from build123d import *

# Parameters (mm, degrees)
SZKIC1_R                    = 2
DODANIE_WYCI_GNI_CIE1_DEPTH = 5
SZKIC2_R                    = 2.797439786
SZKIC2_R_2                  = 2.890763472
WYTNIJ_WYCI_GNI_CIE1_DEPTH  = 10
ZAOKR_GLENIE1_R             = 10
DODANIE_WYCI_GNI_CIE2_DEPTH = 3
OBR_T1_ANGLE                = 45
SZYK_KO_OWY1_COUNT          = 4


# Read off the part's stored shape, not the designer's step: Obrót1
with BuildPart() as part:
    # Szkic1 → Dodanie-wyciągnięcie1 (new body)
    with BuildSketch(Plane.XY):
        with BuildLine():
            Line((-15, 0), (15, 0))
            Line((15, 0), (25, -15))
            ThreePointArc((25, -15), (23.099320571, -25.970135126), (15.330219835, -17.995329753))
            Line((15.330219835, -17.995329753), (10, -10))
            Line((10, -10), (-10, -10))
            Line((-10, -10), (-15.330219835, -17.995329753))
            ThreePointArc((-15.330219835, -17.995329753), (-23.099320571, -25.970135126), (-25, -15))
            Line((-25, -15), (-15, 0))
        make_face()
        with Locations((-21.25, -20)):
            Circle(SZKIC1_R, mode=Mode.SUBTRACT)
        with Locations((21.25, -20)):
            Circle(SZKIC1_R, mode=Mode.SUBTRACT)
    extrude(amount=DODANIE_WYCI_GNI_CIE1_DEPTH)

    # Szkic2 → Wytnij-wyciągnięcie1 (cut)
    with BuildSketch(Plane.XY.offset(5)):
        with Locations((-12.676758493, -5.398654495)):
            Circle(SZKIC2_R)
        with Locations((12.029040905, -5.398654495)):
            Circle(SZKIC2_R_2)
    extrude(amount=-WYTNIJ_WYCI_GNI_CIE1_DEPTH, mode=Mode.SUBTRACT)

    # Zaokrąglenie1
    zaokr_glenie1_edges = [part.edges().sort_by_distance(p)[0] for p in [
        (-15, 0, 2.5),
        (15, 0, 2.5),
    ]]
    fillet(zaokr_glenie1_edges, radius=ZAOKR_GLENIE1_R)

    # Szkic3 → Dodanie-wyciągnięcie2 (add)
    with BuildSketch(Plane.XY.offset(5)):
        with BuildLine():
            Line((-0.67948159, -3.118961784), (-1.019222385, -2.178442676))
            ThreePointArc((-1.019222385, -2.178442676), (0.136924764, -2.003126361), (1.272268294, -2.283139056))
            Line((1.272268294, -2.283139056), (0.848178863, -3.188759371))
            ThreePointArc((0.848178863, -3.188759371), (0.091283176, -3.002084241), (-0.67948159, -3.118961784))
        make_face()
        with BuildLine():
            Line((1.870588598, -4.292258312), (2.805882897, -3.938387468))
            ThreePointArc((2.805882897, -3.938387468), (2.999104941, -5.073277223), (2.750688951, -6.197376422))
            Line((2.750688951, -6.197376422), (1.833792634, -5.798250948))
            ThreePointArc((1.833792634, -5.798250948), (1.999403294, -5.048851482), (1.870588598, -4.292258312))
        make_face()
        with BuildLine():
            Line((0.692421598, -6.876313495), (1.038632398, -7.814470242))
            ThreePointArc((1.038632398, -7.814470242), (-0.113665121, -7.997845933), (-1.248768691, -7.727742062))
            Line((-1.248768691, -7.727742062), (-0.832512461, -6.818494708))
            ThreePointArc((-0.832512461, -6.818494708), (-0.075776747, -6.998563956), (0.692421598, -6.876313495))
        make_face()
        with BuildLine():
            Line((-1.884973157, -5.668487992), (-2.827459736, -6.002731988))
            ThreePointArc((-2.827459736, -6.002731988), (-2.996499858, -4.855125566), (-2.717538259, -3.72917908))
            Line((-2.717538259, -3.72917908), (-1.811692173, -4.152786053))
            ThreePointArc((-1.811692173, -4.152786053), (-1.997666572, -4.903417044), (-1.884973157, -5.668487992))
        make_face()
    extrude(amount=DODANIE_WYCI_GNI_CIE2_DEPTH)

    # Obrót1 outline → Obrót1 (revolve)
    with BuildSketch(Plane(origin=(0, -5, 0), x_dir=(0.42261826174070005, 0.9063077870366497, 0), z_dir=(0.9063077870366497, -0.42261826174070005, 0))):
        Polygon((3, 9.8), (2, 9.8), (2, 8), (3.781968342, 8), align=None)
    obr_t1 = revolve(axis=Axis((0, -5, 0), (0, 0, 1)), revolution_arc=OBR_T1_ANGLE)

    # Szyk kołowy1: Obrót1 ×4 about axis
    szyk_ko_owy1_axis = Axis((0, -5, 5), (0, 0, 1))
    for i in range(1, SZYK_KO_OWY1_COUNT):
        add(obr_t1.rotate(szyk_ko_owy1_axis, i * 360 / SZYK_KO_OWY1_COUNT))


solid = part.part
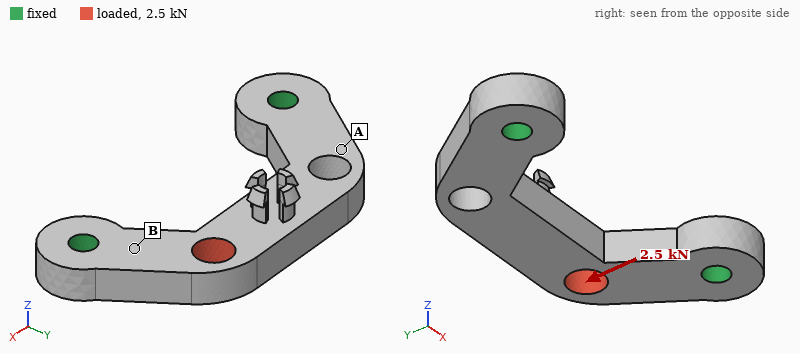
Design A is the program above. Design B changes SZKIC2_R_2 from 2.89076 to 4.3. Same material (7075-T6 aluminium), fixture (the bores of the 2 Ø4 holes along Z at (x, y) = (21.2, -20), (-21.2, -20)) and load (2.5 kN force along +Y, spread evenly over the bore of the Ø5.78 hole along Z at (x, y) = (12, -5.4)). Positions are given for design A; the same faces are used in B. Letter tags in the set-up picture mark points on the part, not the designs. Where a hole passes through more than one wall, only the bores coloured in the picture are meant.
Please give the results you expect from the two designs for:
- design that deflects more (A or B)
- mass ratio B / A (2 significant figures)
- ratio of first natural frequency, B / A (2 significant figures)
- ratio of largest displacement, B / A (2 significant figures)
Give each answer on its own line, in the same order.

B
0.95
0.99
2.0
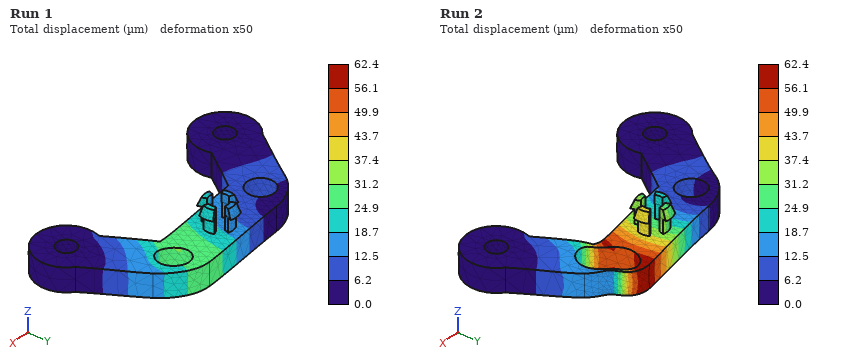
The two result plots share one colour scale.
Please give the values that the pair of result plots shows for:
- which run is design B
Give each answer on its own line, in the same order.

Run 2
